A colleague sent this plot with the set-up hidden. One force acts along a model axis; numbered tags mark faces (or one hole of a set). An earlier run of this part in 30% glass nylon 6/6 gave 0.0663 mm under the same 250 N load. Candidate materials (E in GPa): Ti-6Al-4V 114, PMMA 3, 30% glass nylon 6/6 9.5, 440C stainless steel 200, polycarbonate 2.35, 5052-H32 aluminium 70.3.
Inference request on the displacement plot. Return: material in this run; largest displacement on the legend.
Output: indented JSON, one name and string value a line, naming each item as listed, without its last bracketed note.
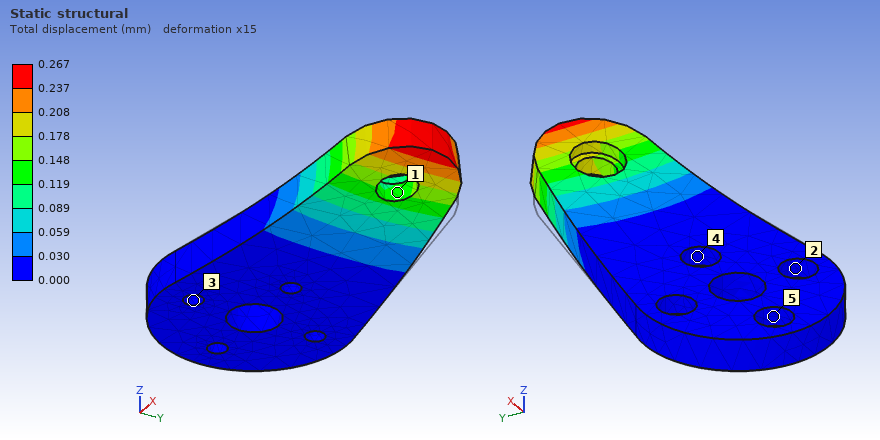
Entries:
{
  "material in this run": "polycarbonate",
  "largest displacement on the legend": "0.267 mm"
}
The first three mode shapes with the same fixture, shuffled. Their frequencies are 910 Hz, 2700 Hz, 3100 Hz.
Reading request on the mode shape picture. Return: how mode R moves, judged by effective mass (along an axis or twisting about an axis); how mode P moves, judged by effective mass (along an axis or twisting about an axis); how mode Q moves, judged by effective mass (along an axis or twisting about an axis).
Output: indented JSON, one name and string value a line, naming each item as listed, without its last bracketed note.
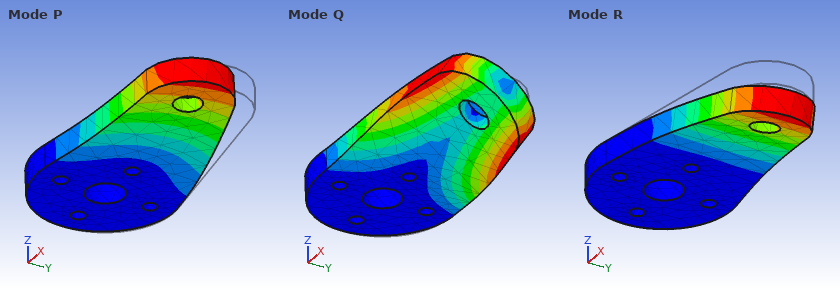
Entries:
{
  "how mode R moves, judged by effective mass": "along Z",
  "how mode P moves, judged by effective mass": "along Y",
  "how mode Q moves, judged by effective mass": "twisting about X"
}
